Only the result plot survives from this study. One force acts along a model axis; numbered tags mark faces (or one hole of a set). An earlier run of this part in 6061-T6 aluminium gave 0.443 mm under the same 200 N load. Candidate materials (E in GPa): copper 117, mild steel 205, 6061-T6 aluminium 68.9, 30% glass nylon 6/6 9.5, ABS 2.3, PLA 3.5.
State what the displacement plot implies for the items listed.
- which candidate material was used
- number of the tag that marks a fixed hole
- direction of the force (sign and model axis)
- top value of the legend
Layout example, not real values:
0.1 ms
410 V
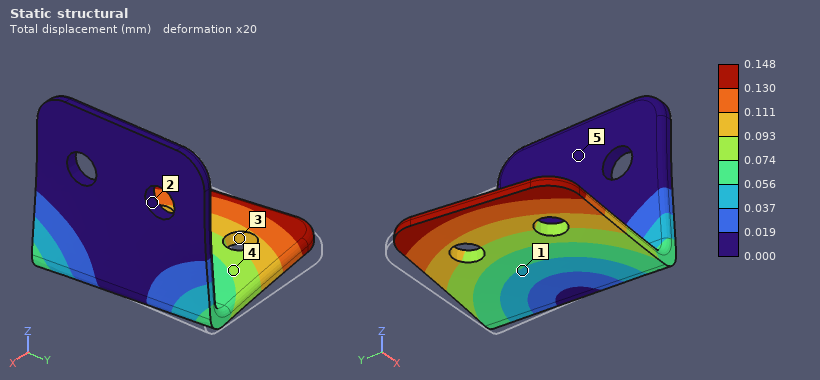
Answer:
mild steel
2
-Y
0.148 mm
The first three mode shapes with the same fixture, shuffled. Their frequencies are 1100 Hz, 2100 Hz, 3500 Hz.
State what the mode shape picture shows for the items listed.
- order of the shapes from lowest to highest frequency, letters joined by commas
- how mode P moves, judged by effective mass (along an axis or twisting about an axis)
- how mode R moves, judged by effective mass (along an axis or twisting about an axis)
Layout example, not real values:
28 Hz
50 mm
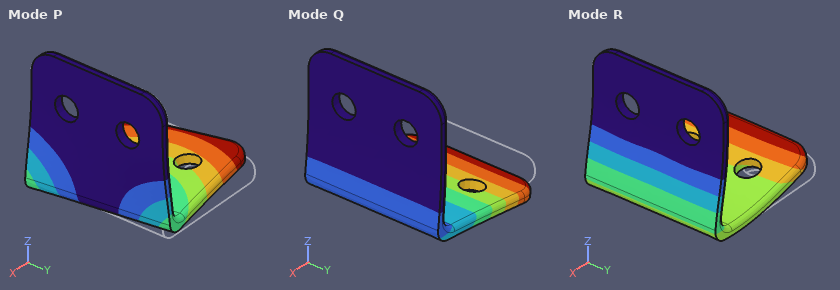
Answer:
Q, P, R
along Y
along X
